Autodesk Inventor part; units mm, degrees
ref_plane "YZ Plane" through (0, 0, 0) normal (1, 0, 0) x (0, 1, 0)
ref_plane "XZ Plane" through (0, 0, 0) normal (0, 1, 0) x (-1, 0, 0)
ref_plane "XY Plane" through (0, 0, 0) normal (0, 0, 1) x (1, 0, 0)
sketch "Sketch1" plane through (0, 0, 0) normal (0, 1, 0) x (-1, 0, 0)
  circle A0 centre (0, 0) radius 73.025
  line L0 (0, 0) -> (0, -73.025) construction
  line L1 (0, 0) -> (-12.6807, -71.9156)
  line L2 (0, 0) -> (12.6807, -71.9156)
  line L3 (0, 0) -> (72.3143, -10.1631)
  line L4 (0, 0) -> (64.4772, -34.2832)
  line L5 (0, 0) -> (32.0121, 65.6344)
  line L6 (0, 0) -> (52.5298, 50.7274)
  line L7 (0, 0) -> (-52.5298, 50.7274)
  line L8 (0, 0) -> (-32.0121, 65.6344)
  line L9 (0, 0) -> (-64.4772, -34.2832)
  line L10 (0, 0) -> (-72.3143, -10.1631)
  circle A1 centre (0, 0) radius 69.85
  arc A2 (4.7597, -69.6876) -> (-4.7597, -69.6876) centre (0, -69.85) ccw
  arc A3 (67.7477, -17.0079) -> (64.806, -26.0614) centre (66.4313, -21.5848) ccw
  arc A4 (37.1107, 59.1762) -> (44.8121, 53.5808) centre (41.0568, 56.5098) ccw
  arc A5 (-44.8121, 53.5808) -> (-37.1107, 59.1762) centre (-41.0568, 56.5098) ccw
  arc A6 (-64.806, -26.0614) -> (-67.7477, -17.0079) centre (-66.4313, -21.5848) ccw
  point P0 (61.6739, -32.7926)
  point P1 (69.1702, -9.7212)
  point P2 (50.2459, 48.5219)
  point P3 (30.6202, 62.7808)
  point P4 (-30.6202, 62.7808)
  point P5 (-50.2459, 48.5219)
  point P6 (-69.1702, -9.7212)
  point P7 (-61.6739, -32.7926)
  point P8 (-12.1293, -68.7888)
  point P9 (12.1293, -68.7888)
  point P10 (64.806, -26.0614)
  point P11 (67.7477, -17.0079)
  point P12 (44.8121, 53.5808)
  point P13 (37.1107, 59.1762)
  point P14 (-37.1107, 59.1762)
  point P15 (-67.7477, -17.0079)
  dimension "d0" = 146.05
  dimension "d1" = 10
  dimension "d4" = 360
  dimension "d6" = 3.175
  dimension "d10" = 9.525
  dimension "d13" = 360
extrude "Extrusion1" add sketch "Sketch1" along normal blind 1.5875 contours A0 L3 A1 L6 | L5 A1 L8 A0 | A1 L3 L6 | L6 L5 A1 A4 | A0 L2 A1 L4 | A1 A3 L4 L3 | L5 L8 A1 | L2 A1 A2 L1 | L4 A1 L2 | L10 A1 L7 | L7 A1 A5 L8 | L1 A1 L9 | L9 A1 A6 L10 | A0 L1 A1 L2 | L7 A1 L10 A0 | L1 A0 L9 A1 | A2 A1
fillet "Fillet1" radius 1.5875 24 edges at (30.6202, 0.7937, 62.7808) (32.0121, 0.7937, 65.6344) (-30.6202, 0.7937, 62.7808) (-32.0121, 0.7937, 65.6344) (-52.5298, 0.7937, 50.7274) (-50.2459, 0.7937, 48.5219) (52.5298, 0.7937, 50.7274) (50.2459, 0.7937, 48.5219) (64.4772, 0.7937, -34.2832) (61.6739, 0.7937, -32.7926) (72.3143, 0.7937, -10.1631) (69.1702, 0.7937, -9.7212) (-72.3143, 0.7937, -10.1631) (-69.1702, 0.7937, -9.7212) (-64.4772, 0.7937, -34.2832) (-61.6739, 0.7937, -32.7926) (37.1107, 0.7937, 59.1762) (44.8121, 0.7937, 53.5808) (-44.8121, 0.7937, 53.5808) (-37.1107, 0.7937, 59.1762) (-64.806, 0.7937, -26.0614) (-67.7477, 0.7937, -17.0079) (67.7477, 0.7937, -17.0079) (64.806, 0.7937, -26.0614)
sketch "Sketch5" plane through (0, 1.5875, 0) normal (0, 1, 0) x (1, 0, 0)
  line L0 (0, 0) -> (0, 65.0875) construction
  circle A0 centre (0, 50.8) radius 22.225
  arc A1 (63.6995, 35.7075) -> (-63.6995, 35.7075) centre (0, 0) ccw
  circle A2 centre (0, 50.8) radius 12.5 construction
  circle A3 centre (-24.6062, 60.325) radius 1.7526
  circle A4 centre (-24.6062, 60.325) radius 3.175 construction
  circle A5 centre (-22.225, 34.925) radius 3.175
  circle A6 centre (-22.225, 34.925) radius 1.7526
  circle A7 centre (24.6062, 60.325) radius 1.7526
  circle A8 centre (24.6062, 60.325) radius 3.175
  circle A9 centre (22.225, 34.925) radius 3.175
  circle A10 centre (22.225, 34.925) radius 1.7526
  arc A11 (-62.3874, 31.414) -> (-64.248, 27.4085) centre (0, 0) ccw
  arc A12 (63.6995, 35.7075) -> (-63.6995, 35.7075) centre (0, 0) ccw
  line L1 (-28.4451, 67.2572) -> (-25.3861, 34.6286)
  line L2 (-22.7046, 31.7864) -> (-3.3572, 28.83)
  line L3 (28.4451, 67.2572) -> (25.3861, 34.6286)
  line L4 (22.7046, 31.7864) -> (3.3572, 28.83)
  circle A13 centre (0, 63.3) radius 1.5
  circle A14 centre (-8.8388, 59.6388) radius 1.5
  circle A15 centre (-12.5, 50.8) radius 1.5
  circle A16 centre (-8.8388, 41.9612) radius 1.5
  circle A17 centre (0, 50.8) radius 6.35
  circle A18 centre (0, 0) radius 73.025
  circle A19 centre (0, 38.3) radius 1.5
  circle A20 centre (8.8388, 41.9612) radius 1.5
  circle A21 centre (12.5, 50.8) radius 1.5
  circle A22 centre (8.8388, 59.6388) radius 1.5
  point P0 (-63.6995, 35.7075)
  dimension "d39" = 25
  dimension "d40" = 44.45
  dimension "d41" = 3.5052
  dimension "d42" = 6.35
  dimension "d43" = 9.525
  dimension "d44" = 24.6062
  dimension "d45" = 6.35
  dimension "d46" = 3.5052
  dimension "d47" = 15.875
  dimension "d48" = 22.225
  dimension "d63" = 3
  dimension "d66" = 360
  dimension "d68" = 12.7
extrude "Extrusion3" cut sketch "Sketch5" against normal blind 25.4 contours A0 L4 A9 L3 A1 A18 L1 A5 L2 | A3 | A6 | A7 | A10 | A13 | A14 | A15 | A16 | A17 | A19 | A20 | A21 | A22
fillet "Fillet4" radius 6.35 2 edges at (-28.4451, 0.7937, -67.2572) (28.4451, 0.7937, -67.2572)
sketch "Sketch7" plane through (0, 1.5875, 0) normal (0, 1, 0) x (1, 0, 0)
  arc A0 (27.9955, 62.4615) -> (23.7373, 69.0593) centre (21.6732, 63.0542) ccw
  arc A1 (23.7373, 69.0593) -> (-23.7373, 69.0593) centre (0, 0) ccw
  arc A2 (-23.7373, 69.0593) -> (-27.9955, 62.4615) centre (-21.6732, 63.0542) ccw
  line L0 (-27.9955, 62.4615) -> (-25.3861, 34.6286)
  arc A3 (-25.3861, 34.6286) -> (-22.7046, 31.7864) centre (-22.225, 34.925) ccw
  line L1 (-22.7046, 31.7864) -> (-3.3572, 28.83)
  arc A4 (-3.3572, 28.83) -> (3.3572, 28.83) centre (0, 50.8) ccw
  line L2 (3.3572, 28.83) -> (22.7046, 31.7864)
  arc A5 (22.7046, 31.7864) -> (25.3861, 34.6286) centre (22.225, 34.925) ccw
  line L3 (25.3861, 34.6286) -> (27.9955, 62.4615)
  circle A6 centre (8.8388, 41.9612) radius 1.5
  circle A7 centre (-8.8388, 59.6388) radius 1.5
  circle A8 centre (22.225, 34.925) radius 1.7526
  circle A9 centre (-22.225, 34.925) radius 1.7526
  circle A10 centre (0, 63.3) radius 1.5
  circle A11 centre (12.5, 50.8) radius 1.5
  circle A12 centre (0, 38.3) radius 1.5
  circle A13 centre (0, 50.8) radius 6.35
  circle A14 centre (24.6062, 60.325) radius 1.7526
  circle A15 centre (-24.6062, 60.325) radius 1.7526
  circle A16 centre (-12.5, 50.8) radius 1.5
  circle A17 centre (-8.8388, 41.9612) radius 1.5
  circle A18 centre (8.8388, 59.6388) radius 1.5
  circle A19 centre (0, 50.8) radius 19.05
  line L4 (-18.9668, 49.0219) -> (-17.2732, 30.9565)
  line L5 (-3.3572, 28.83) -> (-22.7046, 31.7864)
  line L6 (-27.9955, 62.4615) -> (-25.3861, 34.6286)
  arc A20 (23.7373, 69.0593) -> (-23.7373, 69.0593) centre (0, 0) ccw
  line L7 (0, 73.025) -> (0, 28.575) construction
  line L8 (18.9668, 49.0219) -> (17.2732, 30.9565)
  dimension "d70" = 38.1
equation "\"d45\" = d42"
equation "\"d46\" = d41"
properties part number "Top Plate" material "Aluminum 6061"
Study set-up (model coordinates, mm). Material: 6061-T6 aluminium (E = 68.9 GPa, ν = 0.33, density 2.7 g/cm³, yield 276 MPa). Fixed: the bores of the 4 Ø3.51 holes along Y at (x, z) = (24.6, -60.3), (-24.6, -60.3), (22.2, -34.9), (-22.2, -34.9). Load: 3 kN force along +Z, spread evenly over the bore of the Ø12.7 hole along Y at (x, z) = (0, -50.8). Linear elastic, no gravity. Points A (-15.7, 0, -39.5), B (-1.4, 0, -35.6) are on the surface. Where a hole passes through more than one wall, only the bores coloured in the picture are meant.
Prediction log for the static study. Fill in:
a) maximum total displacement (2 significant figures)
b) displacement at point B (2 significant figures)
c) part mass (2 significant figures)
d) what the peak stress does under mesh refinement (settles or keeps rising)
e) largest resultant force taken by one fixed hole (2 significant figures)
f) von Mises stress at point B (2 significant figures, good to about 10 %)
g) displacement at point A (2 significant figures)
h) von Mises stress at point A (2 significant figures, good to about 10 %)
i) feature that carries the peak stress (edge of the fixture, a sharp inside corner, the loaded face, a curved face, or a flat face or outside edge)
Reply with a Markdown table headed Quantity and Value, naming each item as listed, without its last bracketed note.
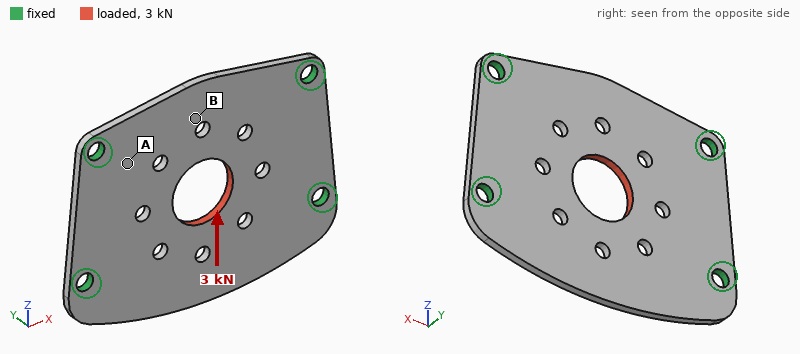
| Quantity | Value |
|---|---|
| maximum total displacement | 31 µm |
| displacement at point B | 24 µm |
| part mass | 8.4 g |
| what the peak stress does under mesh refinement | keeps rising |
| largest resultant force taken by one fixed hole | 910 N |
| von Mises stress at point B | 25 MPa |
| displacement at point A | 9.5 µm |
| von Mises stress at point A | 63 MPa |
| feature that carries the peak stress | edge of the fixture |
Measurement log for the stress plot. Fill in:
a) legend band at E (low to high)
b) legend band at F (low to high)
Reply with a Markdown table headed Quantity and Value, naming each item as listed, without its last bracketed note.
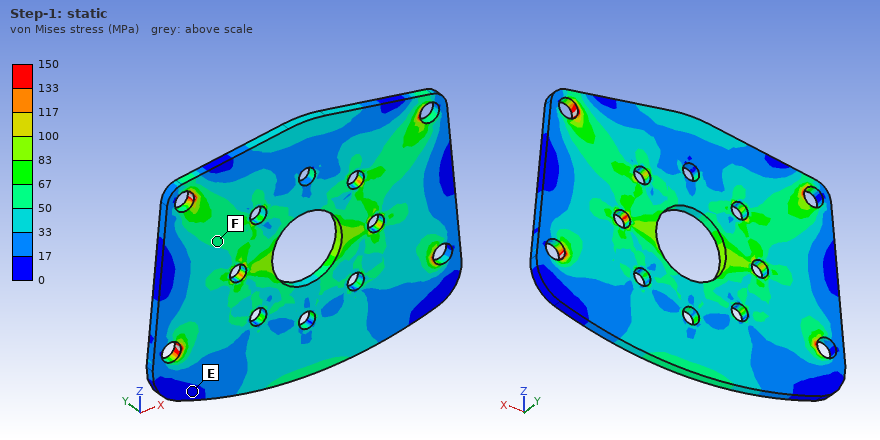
| Quantity | Value |
|---|---|
| legend band at E | 0 to 17 MPa |
| legend band at F | 50 to 67 MPa |
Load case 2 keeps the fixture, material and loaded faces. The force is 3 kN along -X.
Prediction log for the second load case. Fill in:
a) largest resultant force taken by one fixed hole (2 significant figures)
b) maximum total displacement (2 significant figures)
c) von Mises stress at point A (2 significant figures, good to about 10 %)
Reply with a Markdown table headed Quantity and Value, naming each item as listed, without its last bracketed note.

| Quantity | Value |
|---|---|
| largest resultant force taken by one fixed hole | 880 N |
| maximum total displacement | 16 µm |
| von Mises stress at point A | 39 MPa |
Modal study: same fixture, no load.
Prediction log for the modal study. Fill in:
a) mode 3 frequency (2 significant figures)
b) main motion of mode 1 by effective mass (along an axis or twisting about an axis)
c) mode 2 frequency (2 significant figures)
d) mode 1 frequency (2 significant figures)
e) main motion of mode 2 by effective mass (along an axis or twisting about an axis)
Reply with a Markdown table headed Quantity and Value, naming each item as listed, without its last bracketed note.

| Quantity | Value |
|---|---|
| mode 3 frequency | 6800 Hz |
| main motion of mode 1 by effective mass | along Y |
| mode 2 frequency | 4400 Hz |
| mode 1 frequency | 3300 Hz |
| main motion of mode 2 by effective mass | along Y |
